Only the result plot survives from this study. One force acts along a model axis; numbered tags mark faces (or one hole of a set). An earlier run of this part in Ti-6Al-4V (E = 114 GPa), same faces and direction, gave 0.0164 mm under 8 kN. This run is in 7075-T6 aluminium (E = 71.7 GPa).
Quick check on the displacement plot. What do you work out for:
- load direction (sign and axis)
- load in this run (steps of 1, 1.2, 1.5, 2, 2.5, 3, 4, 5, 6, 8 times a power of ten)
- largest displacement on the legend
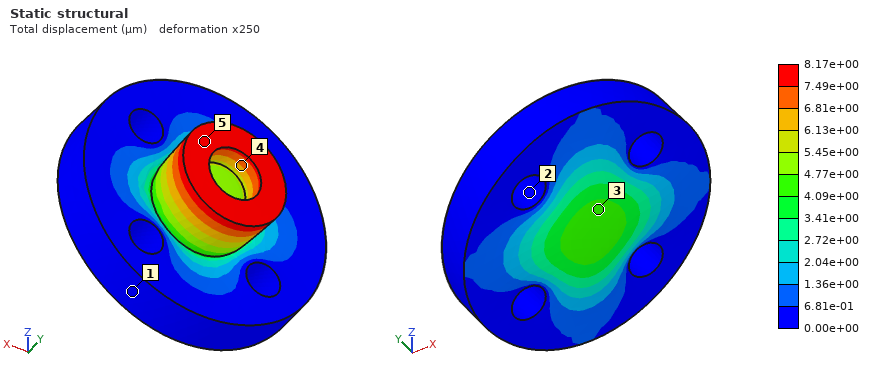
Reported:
-Y
2.5 kN
8.17e+00 µm
